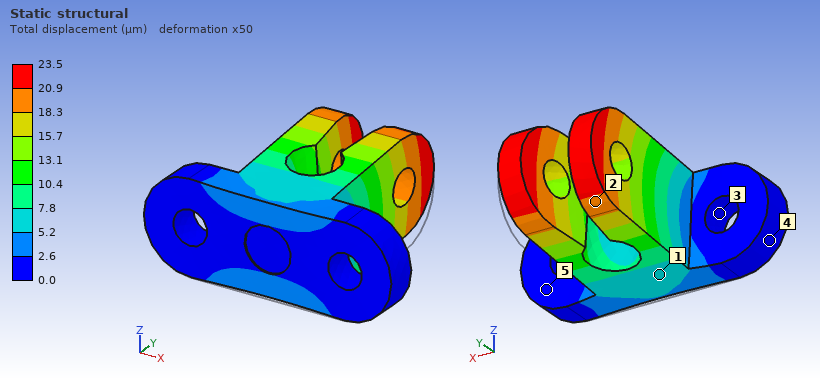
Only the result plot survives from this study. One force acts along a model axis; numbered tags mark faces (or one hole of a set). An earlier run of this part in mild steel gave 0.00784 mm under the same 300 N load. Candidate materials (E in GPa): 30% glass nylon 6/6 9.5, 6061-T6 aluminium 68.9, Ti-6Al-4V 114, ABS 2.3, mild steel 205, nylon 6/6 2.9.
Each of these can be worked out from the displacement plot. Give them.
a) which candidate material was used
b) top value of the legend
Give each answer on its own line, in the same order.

6061-T6 aluminium
23.5 µm
